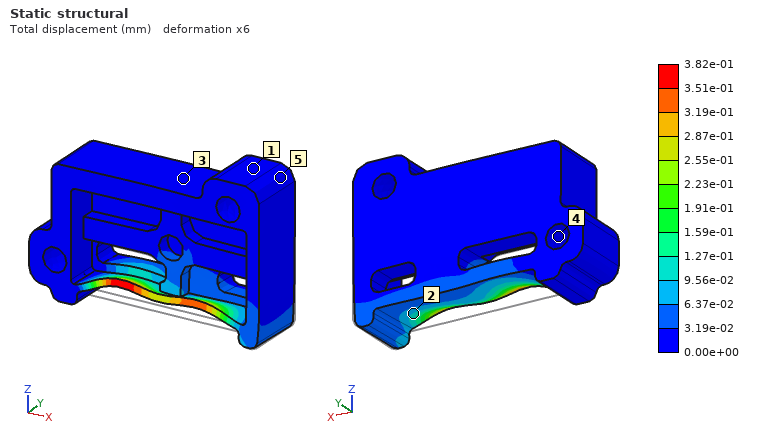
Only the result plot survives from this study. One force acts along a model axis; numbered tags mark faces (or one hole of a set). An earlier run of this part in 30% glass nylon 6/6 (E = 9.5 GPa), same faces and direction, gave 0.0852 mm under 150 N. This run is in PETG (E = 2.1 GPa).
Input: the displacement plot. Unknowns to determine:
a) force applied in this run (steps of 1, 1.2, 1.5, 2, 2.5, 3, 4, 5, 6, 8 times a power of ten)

150 N
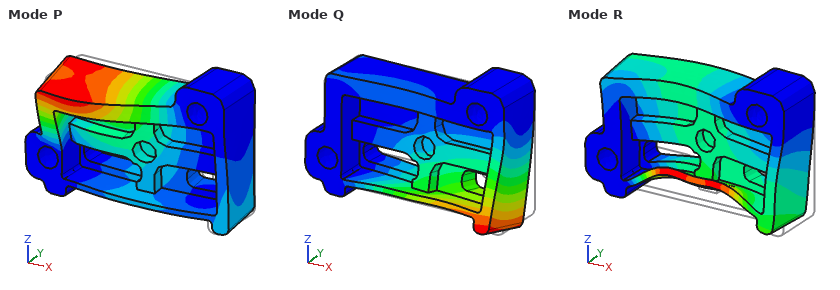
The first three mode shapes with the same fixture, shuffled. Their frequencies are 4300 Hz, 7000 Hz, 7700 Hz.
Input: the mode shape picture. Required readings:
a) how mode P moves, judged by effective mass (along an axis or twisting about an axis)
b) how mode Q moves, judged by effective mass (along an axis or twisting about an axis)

along Y
along Y
